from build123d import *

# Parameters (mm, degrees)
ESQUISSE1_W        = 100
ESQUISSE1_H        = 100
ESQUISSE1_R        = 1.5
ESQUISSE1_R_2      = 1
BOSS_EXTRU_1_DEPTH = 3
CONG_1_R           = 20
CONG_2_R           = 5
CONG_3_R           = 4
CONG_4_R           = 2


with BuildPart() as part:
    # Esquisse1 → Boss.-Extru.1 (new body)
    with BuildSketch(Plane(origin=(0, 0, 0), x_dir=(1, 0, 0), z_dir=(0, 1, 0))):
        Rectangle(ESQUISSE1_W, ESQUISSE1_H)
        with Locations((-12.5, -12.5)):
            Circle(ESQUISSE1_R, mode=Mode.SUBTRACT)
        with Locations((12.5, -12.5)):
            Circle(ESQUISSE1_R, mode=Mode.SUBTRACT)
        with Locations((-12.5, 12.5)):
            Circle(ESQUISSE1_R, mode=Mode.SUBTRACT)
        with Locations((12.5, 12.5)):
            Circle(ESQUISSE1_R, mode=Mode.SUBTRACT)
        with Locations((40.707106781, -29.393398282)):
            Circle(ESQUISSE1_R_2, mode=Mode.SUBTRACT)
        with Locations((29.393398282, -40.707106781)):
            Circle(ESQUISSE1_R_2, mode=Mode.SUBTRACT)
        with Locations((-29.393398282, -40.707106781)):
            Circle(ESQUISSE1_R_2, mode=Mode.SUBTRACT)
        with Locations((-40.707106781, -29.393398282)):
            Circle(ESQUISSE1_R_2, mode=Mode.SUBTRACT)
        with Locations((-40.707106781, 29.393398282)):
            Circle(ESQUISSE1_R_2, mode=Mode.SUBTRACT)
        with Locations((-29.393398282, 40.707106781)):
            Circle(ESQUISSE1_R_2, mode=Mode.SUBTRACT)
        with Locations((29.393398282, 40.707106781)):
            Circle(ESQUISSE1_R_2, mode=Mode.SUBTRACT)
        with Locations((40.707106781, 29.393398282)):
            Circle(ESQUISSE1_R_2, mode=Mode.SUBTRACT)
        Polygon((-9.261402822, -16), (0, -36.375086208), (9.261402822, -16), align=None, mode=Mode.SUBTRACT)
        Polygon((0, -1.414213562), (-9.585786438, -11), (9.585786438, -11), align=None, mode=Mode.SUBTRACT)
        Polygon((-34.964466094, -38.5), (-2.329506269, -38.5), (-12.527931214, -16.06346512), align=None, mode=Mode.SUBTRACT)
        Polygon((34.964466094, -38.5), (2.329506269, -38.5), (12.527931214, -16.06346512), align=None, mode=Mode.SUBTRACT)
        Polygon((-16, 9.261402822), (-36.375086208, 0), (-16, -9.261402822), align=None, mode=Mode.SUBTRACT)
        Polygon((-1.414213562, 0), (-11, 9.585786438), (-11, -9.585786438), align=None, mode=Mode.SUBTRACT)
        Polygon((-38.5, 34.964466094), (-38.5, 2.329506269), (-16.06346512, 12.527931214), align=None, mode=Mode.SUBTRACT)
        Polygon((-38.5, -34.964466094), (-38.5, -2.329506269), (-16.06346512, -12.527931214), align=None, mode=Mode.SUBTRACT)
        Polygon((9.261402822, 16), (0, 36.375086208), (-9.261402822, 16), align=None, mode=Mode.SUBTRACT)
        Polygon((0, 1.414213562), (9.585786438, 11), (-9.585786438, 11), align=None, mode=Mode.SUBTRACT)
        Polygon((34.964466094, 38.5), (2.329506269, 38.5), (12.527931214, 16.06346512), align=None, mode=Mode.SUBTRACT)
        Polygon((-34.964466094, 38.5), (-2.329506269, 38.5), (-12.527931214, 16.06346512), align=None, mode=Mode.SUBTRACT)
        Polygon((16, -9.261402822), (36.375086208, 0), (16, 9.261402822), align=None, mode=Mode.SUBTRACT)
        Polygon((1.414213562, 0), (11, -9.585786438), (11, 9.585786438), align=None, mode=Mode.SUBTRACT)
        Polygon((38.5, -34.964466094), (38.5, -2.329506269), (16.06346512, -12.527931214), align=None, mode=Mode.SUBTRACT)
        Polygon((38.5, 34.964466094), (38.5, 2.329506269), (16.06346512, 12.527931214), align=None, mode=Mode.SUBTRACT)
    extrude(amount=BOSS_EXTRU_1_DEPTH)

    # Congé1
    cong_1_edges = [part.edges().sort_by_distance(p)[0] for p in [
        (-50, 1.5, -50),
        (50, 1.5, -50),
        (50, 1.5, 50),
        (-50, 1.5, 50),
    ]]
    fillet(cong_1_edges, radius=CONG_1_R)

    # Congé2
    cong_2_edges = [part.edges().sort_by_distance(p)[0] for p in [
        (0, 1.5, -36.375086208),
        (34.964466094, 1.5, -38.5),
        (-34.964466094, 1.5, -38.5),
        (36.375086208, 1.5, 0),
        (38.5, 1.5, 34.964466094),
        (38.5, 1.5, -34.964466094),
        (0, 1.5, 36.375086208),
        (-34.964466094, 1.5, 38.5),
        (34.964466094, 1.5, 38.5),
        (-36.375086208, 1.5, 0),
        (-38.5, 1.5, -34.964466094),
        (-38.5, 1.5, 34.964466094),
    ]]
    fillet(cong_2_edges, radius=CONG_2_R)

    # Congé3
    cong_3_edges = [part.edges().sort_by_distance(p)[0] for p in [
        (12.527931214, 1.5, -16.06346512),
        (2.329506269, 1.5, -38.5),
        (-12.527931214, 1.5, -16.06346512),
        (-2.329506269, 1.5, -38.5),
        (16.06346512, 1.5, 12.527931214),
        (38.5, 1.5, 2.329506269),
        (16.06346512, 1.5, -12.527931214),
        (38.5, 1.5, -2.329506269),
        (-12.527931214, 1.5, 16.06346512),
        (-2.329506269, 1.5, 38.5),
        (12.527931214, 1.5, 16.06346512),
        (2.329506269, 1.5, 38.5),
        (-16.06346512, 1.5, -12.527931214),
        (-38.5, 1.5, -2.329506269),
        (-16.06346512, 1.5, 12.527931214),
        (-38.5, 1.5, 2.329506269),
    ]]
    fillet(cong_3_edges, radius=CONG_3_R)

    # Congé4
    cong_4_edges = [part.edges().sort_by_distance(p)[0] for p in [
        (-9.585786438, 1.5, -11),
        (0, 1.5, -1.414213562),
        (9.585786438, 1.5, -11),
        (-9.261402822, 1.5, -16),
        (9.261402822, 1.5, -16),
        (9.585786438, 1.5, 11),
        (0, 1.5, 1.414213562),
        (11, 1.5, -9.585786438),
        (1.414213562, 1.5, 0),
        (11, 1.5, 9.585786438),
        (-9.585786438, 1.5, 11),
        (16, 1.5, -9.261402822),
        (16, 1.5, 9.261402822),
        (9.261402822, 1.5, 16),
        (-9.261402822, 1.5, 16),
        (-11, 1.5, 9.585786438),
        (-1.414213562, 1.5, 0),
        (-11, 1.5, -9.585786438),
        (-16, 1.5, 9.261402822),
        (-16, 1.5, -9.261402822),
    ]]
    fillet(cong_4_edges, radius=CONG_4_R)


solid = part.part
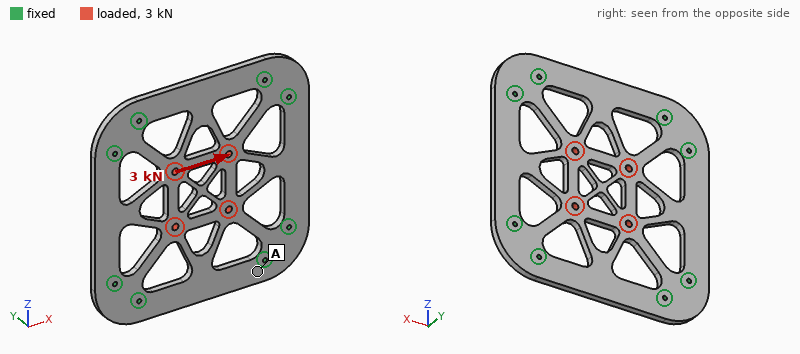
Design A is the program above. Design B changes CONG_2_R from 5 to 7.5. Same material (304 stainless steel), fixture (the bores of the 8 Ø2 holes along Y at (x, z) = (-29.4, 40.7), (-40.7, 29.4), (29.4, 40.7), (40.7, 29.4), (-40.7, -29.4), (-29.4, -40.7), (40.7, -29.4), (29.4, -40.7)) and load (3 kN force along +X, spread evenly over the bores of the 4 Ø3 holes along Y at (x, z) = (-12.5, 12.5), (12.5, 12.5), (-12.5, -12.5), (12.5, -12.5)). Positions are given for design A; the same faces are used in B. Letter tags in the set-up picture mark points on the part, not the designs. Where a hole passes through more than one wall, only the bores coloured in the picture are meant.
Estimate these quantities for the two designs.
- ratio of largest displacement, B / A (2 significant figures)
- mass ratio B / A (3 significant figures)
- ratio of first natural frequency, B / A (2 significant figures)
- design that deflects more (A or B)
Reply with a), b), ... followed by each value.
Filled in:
a) 0.84
b) 1.07
c) 1.1
d) A
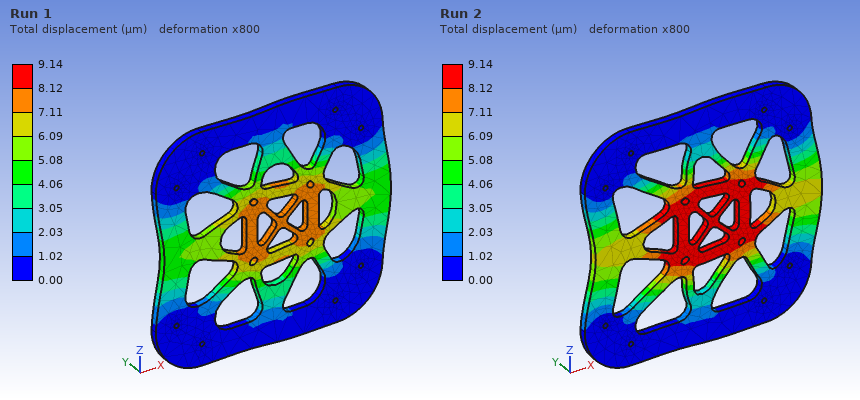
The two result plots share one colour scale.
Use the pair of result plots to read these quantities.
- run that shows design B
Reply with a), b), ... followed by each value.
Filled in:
a) Run 1
